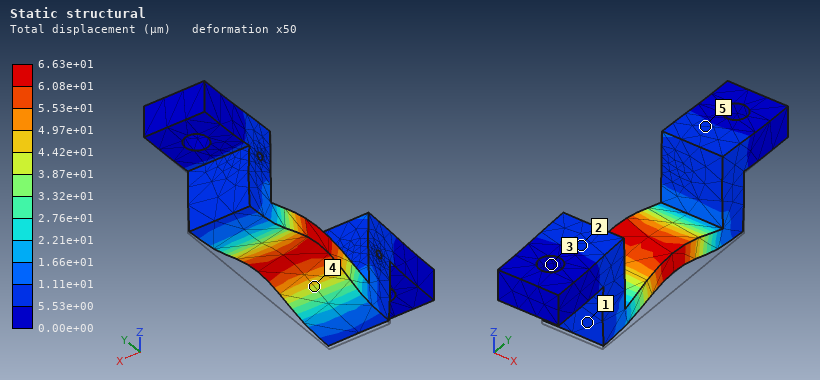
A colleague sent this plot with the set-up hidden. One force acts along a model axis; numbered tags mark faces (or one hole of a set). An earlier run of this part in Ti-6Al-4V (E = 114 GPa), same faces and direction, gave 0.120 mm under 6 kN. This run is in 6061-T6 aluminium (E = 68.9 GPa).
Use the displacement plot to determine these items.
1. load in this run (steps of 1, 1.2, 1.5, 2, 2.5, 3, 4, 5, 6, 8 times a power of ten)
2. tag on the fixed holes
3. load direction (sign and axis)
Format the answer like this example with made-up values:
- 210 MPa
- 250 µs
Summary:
- 2 kN
- 3
- +Z
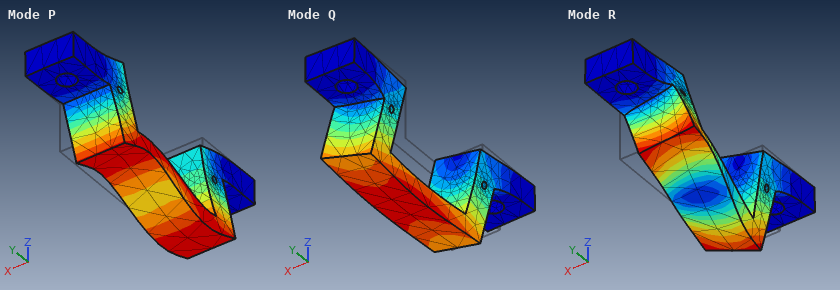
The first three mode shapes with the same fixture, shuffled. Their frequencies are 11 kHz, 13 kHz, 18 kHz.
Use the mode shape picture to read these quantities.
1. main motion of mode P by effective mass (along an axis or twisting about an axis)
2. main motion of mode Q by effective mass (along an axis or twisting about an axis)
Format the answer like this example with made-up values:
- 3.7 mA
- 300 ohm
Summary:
- along Y
- along X
